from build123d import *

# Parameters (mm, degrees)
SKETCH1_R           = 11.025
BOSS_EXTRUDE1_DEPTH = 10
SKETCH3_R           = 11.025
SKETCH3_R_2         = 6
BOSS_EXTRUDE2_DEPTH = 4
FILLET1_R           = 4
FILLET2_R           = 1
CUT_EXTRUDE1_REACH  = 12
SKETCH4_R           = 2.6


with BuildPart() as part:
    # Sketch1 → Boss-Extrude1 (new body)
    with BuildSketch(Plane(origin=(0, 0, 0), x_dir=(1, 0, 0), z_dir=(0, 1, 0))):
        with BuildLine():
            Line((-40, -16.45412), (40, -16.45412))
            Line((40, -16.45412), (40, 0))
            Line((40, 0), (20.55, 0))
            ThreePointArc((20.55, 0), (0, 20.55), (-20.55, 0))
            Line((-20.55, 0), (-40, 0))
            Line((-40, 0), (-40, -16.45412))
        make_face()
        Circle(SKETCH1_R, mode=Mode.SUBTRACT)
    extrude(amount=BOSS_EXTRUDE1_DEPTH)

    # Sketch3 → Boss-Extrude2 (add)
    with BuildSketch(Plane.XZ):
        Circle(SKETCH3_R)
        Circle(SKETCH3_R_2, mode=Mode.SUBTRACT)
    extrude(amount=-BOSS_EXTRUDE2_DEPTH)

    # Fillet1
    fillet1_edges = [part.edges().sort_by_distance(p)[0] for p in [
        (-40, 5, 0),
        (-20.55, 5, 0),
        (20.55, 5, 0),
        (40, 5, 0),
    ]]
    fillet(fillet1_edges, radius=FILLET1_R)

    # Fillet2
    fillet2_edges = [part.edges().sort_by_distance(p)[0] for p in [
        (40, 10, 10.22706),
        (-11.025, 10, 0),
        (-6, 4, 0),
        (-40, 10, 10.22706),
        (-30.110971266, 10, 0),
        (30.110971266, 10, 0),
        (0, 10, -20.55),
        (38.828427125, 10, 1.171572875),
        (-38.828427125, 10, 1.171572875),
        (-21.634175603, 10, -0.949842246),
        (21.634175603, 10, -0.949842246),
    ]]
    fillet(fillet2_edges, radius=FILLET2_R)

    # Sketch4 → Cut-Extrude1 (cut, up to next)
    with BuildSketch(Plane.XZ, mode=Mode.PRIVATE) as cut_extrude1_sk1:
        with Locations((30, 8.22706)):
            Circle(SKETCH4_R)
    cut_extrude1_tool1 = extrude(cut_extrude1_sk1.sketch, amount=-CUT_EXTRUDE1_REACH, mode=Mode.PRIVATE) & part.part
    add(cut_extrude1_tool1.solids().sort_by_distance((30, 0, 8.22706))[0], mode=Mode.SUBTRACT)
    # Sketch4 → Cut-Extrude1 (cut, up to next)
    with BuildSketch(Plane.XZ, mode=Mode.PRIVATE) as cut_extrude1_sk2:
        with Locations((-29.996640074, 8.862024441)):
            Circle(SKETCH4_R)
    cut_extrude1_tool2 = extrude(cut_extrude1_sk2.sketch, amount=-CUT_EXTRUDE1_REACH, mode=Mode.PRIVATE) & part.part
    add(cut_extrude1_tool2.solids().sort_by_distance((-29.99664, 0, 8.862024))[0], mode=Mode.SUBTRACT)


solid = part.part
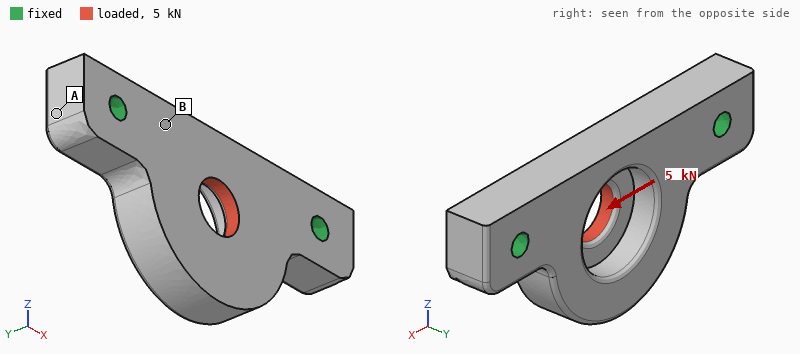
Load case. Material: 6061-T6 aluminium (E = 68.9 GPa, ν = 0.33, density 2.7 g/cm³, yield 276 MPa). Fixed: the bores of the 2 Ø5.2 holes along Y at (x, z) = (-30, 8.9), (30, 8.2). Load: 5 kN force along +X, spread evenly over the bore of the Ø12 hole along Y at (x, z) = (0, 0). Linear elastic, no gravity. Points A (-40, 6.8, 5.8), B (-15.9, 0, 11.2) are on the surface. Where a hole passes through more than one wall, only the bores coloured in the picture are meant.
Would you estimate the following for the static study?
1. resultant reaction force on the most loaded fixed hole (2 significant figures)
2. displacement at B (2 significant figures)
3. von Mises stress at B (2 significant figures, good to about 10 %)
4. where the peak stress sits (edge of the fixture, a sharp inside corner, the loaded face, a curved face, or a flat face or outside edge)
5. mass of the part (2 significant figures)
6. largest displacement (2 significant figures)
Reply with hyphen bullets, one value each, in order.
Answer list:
- 2.6 kN
- 2.6 µm
- 16 MPa
- the loaded face
- 45 g
- 15 µm
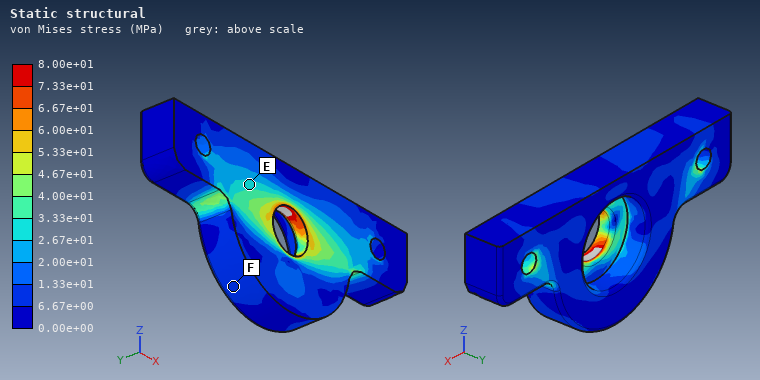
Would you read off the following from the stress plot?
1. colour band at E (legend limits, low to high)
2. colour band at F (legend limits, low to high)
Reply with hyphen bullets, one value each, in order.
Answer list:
- 2.67e+01 to 3.33e+01 MPa
- 6.67e+00 to 1.33e+01 MPa
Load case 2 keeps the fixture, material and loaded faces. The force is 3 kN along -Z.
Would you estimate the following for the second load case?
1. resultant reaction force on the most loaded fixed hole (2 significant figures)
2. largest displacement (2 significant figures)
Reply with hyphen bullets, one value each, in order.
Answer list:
- 1.5 kN
- 40 µm
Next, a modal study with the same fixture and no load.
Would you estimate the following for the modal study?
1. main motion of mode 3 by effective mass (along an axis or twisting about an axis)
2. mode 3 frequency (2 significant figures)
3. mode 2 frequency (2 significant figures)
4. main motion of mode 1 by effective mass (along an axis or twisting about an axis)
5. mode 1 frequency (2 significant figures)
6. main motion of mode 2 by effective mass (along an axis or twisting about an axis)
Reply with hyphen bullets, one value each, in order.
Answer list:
- along Z
- 16 kHz
- 14 kHz
- along Y
- 6300 Hz
- along Y
